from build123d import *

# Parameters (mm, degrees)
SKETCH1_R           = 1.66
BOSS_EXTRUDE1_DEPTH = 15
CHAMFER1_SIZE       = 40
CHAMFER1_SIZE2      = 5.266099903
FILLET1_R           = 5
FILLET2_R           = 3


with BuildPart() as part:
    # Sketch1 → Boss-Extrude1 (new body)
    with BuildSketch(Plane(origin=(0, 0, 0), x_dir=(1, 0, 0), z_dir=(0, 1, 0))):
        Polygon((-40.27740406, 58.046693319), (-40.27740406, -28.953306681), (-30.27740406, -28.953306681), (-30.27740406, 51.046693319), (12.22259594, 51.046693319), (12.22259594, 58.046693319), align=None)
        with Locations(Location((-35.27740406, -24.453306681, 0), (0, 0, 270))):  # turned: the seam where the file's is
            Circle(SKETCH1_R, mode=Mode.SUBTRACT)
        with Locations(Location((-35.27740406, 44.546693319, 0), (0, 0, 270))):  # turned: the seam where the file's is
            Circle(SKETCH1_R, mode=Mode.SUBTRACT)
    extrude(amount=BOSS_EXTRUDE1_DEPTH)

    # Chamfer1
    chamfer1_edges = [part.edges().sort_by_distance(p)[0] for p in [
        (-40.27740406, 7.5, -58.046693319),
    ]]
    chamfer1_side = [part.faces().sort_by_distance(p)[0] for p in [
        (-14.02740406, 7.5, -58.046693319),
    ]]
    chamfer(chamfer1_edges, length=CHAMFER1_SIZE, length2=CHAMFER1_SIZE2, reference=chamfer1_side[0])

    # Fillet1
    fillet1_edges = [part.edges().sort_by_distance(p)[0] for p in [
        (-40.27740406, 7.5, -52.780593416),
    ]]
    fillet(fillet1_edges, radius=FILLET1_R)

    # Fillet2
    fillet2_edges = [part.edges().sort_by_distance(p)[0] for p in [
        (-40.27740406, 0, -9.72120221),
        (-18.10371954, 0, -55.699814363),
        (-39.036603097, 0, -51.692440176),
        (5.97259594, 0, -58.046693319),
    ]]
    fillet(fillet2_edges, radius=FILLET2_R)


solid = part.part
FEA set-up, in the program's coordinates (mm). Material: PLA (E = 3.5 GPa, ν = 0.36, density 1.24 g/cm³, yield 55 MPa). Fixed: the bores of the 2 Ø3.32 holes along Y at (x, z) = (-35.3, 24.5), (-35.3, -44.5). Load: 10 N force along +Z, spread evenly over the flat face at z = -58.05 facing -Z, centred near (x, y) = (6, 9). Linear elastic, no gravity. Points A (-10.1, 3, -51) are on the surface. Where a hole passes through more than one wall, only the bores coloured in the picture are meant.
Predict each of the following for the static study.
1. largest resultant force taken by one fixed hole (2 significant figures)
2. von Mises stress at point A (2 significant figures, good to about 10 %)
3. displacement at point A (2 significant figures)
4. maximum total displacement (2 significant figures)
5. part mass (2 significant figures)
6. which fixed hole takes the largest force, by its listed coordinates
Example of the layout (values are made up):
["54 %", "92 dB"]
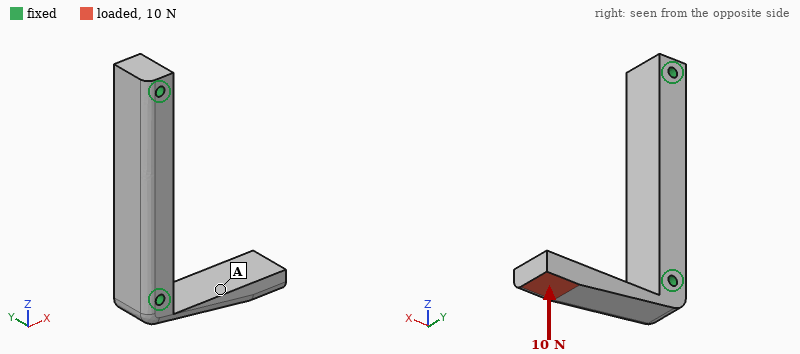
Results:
["9.7 N", "2.1 MPa", "0.42 mm", "1.1 mm", "19 g", "(-35.3, -44.5)"]
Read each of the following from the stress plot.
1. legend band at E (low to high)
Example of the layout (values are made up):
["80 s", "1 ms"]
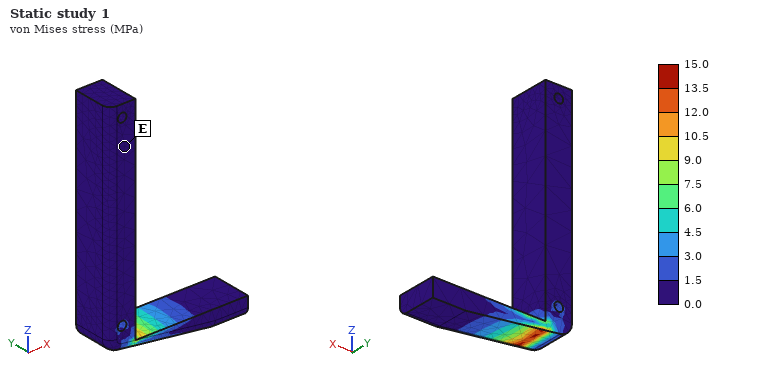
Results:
["0.0 to 1.5 MPa"]
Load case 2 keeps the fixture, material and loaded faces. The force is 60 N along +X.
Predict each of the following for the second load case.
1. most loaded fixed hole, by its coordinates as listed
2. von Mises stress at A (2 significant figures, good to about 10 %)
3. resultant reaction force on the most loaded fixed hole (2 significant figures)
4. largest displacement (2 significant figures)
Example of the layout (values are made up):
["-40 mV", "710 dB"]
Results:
["(-35.3, -44.5)", "2.7 MPa", "63 N", "1.1 mm"]
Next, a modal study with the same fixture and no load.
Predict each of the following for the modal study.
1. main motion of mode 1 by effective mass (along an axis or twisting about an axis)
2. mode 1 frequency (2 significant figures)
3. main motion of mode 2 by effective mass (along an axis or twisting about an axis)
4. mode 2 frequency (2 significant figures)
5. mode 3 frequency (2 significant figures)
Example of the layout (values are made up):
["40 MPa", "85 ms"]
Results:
["along Z", "360 Hz", "along Y", "1000 Hz", "2500 Hz"]
